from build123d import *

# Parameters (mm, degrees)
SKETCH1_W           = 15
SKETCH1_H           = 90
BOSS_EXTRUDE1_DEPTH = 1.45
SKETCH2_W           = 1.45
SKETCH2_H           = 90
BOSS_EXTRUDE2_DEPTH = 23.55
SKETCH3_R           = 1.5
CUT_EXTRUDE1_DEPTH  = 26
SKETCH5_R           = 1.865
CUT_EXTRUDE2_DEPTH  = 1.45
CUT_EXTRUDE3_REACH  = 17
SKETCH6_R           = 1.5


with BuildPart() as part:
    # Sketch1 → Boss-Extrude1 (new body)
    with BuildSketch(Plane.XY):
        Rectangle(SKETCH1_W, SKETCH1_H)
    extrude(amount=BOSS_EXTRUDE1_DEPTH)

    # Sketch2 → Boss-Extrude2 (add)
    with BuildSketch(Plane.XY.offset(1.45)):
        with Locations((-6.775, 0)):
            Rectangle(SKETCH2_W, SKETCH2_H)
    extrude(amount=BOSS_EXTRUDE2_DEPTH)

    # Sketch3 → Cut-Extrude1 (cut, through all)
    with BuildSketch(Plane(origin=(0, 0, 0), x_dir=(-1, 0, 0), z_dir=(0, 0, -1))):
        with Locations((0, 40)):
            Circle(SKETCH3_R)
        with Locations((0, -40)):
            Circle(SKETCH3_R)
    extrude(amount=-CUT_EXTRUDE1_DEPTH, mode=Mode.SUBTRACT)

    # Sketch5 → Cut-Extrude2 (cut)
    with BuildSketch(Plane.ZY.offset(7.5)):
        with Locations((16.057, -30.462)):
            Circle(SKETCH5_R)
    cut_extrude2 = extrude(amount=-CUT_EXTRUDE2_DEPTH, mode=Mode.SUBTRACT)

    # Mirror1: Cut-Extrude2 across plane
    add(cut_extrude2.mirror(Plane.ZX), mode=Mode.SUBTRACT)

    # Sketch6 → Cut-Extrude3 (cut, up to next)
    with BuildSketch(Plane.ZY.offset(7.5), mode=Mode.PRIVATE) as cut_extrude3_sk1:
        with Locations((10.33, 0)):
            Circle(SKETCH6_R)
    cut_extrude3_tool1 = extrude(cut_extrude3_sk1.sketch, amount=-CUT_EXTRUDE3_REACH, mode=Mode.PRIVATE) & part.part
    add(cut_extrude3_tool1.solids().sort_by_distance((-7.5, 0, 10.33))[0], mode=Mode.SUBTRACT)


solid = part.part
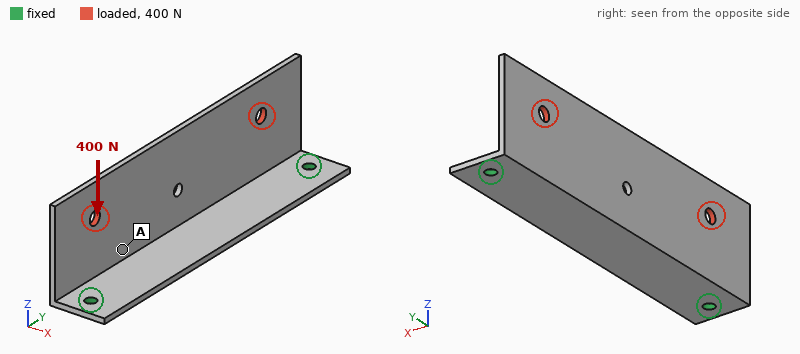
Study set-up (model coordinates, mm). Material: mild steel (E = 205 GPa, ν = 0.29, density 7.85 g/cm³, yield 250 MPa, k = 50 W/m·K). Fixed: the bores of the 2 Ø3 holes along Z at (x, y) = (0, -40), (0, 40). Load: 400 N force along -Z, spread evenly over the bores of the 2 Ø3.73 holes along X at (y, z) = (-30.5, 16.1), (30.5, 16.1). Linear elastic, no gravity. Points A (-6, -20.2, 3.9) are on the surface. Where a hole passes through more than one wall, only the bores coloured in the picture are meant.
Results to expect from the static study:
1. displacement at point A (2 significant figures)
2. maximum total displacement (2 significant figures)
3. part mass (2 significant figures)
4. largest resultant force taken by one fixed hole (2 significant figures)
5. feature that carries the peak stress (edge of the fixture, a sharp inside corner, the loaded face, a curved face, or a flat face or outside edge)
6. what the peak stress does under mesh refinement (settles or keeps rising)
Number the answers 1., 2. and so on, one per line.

1. 0.027 mm
2. 0.11 mm
3. 39 g
4. 210 N
5. edge of the fixture
6. keeps rising
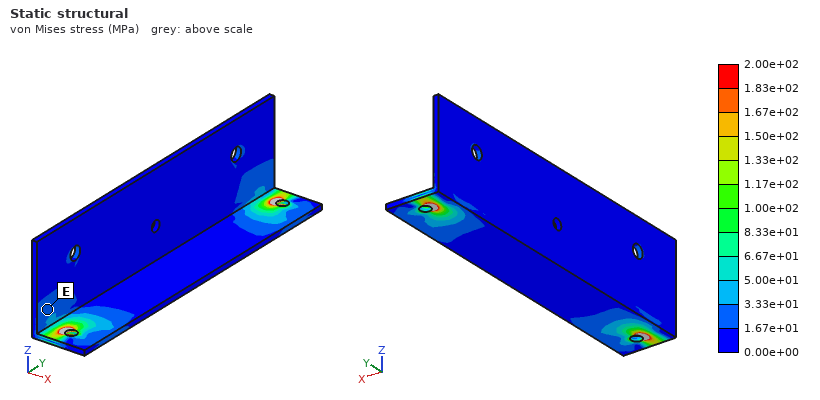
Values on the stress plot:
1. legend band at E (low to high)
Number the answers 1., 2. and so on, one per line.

1. 1.67e+01 to 3.33e+01 MPa
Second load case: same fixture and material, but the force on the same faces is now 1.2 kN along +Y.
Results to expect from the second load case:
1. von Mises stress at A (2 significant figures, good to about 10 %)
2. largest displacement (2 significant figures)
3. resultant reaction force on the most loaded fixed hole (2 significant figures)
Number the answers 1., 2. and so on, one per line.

1. 35 MPa
2. 88 µm
3. 650 N
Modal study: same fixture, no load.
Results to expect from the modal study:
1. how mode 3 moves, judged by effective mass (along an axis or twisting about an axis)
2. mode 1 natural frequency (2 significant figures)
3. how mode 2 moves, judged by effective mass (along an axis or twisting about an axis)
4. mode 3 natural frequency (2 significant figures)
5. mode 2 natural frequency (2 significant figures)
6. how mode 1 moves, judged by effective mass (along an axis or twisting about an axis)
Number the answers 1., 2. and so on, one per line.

1. along Z
2. 990 Hz
3. twisting about Z
4. 2600 Hz
5. 1800 Hz
6. along X
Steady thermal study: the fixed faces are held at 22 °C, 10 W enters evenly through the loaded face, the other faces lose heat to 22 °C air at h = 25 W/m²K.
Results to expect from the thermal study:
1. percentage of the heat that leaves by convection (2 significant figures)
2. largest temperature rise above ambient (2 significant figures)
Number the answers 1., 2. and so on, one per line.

1. 47 %
2. 57 K
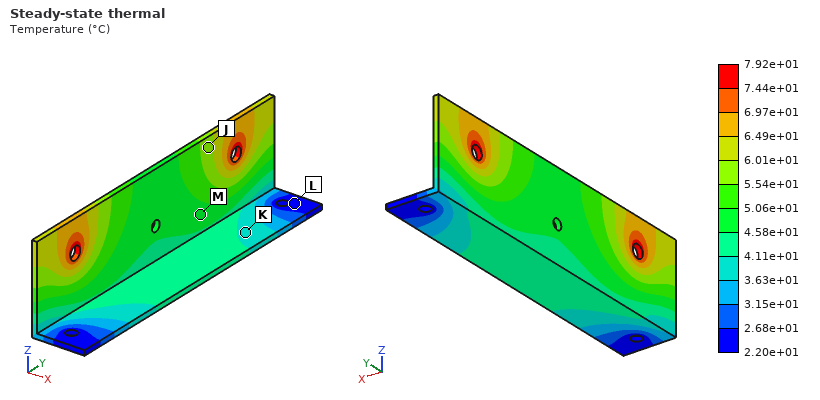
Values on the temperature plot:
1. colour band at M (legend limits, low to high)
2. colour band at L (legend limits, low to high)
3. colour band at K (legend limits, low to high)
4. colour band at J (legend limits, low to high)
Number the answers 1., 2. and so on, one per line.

1. 4.58e+01 to 5.06e+01 °C
2. 2.20e+01 to 2.68e+01 °C
3. 3.63e+01 to 4.11e+01 °C
4. 5.54e+01 to 6.01e+01 °C
